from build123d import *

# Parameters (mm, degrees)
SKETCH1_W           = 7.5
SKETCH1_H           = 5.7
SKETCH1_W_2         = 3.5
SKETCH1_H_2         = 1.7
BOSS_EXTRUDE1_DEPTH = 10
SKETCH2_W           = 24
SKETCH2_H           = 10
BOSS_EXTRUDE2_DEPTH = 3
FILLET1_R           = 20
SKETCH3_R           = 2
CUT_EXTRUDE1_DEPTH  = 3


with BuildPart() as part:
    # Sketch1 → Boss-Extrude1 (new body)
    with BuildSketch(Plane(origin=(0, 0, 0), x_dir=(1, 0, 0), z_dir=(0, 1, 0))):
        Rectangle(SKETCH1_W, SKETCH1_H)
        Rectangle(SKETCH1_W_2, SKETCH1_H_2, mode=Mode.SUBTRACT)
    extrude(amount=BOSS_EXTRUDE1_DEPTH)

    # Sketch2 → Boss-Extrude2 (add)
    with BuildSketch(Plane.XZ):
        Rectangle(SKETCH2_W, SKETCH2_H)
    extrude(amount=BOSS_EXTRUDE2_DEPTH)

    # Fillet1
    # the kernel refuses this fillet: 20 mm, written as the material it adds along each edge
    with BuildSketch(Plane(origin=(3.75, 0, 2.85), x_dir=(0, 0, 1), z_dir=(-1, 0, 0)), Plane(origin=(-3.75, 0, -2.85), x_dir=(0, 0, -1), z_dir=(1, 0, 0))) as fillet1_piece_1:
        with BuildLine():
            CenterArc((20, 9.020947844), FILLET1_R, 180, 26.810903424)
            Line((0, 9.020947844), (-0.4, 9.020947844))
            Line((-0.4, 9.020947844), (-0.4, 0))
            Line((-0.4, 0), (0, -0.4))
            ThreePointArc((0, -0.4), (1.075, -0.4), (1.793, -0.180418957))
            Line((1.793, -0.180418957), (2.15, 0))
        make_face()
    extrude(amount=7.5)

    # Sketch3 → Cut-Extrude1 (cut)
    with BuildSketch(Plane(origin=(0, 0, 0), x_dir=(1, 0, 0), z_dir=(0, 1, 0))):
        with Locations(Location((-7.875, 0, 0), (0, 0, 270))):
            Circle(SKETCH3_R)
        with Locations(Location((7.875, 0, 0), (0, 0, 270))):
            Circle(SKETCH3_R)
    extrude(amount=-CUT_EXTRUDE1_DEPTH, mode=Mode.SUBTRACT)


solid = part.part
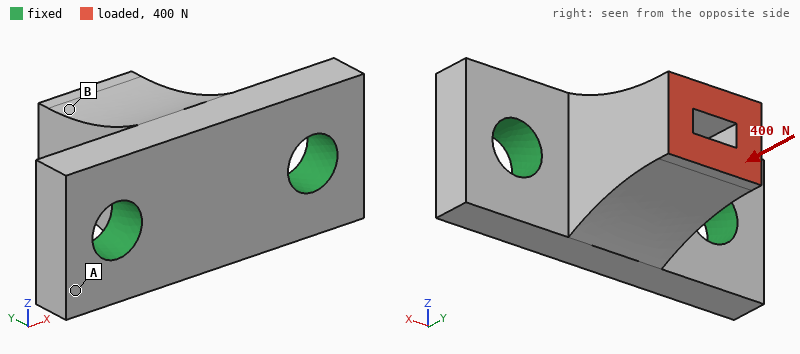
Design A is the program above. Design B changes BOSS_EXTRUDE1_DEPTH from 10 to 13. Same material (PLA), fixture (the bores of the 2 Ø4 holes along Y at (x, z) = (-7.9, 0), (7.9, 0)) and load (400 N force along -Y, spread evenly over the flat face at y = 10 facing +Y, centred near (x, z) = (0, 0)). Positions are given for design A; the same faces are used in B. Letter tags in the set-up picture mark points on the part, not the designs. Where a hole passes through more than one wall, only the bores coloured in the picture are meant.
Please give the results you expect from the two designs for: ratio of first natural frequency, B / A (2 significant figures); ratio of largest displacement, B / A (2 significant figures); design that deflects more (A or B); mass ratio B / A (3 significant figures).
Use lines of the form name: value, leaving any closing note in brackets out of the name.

ratio of first natural frequency, B / A: 0.74
ratio of largest displacement, B / A: 1.1
design that deflects more: B
mass ratio B / A: 1.10
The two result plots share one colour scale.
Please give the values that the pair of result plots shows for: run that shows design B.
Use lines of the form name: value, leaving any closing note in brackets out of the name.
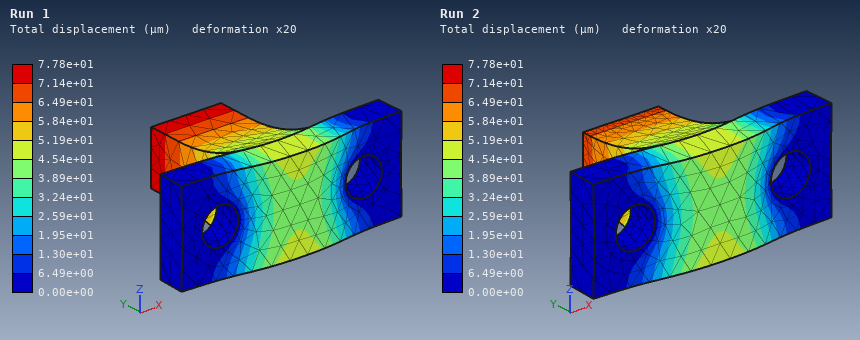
run that shows design B: Run 1
